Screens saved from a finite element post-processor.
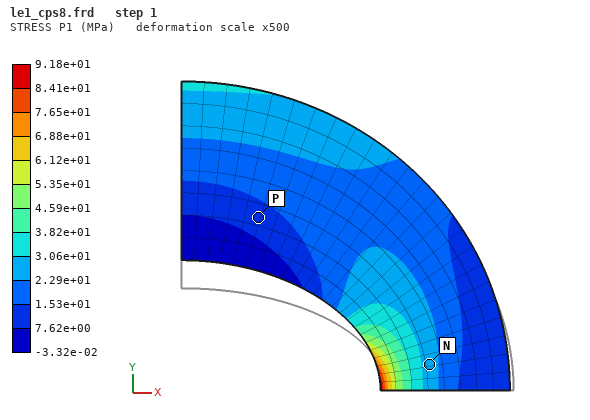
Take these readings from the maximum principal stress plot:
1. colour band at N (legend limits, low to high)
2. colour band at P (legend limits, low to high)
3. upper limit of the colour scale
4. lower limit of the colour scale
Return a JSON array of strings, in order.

["2.29e+01 to 3.06e+01 MPa", "7.62e+00 to 1.53e+01 MPa", "9.18e+01 MPa", "-3.32e-02 MPa"]
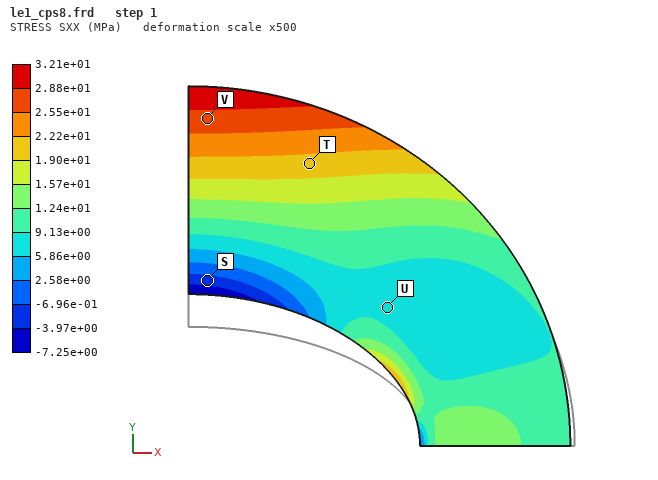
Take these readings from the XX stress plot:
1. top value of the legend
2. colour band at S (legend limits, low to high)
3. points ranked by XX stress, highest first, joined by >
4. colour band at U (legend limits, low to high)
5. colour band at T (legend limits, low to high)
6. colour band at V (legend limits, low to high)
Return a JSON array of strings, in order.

["3.21e+01 MPa", "-3.97e+00 to -6.96e-01 MPa", "V > T > U > S", "5.86e+00 to 9.13e+00 MPa", "1.90e+01 to 2.22e+01 MPa", "2.55e+01 to 2.88e+01 MPa"]
